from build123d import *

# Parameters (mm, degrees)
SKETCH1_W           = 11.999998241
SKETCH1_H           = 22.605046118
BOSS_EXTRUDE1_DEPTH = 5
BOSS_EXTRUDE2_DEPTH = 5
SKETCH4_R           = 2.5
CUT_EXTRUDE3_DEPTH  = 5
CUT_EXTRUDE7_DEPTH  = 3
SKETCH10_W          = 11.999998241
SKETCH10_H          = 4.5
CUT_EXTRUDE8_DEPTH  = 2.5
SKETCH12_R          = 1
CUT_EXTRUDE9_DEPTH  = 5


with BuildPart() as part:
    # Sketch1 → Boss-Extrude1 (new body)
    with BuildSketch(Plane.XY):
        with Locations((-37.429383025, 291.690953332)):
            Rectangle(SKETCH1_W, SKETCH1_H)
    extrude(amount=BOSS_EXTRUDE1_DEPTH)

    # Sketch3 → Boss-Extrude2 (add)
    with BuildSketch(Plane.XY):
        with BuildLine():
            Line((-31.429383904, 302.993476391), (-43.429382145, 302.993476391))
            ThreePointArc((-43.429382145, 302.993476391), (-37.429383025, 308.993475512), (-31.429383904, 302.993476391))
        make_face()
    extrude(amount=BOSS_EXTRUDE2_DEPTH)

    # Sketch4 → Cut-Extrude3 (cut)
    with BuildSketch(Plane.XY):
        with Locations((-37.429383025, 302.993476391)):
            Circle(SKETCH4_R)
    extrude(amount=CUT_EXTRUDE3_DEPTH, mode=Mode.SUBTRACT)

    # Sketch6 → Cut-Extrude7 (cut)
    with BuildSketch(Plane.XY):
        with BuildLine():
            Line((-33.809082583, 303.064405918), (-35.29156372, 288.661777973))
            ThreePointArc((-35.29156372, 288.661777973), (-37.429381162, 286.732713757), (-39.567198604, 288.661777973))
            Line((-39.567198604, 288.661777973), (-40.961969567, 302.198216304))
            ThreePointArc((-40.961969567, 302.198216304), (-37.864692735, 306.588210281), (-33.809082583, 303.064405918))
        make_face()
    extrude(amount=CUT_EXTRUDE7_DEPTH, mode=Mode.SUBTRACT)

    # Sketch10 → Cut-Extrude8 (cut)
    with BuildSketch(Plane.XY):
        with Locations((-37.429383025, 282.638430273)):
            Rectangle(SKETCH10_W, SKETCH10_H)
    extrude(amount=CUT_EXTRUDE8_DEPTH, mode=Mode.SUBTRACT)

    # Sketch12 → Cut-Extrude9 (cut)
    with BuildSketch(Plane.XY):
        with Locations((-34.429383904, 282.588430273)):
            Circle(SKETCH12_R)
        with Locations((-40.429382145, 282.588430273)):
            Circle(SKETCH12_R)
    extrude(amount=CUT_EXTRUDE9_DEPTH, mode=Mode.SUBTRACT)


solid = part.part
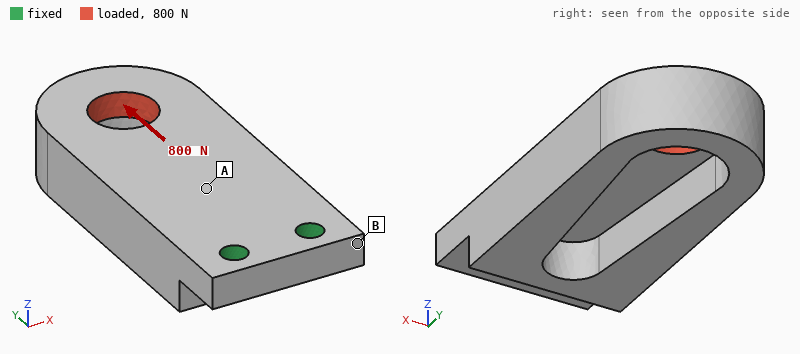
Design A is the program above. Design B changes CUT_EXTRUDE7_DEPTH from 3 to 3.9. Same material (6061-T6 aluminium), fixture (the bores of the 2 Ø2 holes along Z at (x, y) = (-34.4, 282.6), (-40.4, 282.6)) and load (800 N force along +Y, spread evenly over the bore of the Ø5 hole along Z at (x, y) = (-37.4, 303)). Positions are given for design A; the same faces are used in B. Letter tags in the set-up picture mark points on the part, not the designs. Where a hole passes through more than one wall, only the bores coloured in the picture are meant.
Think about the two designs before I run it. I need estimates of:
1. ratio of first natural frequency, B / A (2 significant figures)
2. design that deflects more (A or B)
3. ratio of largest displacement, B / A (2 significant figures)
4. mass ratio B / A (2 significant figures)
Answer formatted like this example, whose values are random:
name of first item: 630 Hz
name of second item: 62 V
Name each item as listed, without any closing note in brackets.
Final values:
ratio of first natural frequency, B / A: 1.0
design that deflects more: B
ratio of largest displacement, B / A: 1.8
mass ratio B / A: 0.93
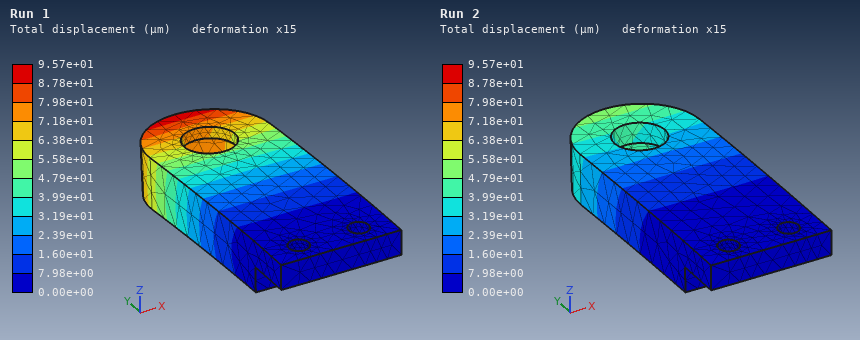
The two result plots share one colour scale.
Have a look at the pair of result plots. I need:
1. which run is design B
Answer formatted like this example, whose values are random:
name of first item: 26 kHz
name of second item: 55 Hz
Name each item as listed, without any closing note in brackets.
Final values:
which run is design B: Run 1
